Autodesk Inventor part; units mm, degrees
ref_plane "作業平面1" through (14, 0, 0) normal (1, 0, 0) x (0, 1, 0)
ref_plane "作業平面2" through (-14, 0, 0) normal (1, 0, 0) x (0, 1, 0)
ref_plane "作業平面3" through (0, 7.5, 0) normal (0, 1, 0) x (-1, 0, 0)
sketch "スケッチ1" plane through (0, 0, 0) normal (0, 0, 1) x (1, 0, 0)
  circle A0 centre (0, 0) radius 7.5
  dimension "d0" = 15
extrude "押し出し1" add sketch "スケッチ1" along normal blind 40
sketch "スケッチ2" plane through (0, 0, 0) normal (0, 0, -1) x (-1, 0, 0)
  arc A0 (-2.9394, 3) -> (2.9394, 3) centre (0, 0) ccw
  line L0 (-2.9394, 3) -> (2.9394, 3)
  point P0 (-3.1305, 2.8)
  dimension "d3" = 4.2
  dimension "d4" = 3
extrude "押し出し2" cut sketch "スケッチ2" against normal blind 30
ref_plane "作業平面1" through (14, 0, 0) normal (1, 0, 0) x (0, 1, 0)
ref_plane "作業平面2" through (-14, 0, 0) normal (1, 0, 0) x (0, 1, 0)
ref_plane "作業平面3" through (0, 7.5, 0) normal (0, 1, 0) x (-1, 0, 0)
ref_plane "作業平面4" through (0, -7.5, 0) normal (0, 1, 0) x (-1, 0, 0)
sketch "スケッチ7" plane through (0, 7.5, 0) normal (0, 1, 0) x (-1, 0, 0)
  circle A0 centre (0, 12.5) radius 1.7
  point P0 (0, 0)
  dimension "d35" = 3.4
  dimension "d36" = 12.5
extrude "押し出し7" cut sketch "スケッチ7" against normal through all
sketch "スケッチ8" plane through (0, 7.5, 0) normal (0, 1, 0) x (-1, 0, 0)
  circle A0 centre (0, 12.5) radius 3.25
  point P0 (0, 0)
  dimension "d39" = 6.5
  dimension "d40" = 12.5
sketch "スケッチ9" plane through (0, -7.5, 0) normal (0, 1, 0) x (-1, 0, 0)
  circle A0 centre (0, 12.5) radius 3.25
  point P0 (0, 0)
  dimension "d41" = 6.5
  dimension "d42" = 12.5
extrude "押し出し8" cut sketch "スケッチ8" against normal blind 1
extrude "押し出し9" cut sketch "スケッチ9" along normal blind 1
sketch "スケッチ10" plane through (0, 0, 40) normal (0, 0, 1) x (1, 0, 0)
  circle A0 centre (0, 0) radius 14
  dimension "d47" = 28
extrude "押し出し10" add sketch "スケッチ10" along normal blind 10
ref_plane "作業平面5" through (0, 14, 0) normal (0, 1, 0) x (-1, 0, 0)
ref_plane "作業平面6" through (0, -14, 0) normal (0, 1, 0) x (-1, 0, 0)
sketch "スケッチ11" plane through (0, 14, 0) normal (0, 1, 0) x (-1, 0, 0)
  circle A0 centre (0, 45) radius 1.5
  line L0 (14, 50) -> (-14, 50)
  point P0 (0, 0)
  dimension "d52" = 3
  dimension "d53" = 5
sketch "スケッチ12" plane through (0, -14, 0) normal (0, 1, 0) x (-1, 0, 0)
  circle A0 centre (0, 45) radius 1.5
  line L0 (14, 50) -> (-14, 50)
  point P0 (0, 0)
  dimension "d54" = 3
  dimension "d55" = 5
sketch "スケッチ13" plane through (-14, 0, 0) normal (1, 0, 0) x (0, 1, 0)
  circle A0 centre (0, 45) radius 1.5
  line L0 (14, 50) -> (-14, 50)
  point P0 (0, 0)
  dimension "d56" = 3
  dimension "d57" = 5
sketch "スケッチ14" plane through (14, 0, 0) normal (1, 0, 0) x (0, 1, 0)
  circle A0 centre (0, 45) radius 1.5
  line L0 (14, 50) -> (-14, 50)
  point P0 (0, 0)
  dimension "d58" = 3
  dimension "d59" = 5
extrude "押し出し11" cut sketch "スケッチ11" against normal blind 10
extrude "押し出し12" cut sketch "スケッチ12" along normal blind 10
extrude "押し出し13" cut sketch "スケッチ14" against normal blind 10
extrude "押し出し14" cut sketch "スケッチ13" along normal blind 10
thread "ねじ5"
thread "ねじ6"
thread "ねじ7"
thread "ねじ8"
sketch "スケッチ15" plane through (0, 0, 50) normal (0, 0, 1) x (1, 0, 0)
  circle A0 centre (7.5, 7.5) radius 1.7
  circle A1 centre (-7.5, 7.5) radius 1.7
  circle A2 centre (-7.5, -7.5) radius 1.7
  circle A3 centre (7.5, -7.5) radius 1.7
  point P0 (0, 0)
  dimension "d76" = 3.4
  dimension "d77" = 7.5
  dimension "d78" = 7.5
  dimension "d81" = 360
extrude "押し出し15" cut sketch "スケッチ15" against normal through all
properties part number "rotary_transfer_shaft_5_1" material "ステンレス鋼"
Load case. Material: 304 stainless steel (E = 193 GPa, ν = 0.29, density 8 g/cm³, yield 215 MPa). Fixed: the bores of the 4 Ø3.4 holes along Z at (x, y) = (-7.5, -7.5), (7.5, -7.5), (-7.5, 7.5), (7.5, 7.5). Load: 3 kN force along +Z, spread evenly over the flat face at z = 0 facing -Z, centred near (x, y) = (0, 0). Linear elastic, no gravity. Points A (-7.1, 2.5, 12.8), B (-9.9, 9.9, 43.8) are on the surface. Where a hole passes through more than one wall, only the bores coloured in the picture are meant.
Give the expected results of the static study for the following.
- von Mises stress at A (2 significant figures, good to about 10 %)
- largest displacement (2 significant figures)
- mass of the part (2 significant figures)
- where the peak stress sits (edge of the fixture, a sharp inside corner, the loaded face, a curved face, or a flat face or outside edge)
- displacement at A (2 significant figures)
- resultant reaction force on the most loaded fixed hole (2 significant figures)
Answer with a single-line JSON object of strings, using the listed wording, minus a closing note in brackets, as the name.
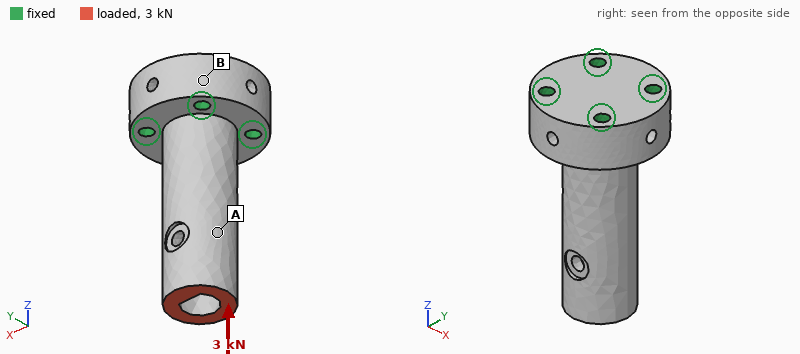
{"von Mises stress at A": "22 MPa", "largest displacement": "5.9 µm", "mass of the part": "88 g", "where the peak stress sits": "a curved face", "displacement at A": "4.0 µm", "resultant reaction force on the most loaded fixed hole": "800 N"}
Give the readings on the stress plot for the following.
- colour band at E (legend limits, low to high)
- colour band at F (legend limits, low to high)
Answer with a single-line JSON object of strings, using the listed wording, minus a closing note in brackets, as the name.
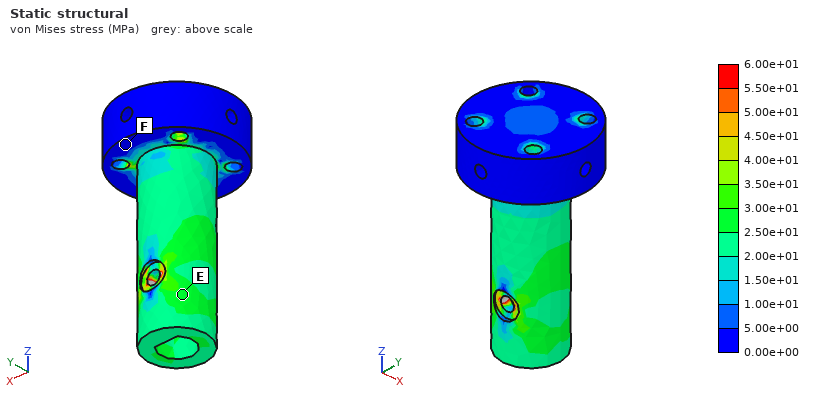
{"colour band at E": "2.50e+01 to 3.00e+01 MPa", "colour band at F": "0.00e+00 to 5.00e+00 MPa"}
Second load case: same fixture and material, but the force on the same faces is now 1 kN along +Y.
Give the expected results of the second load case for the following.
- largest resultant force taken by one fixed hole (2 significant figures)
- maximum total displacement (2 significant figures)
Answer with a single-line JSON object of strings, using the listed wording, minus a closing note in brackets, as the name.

{"largest resultant force taken by one fixed hole": "1.5 kN", "maximum total displacement": "70 µm"}
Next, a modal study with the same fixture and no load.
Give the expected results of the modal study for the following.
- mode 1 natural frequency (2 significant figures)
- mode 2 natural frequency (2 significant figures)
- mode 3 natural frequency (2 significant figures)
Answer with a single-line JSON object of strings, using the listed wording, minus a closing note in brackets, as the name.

{"mode 1 natural frequency": "5900 Hz", "mode 2 natural frequency": "5900 Hz", "mode 3 natural frequency": "19 kHz"}
